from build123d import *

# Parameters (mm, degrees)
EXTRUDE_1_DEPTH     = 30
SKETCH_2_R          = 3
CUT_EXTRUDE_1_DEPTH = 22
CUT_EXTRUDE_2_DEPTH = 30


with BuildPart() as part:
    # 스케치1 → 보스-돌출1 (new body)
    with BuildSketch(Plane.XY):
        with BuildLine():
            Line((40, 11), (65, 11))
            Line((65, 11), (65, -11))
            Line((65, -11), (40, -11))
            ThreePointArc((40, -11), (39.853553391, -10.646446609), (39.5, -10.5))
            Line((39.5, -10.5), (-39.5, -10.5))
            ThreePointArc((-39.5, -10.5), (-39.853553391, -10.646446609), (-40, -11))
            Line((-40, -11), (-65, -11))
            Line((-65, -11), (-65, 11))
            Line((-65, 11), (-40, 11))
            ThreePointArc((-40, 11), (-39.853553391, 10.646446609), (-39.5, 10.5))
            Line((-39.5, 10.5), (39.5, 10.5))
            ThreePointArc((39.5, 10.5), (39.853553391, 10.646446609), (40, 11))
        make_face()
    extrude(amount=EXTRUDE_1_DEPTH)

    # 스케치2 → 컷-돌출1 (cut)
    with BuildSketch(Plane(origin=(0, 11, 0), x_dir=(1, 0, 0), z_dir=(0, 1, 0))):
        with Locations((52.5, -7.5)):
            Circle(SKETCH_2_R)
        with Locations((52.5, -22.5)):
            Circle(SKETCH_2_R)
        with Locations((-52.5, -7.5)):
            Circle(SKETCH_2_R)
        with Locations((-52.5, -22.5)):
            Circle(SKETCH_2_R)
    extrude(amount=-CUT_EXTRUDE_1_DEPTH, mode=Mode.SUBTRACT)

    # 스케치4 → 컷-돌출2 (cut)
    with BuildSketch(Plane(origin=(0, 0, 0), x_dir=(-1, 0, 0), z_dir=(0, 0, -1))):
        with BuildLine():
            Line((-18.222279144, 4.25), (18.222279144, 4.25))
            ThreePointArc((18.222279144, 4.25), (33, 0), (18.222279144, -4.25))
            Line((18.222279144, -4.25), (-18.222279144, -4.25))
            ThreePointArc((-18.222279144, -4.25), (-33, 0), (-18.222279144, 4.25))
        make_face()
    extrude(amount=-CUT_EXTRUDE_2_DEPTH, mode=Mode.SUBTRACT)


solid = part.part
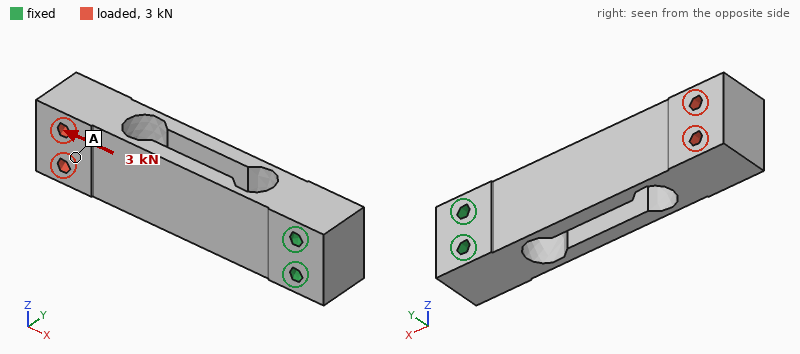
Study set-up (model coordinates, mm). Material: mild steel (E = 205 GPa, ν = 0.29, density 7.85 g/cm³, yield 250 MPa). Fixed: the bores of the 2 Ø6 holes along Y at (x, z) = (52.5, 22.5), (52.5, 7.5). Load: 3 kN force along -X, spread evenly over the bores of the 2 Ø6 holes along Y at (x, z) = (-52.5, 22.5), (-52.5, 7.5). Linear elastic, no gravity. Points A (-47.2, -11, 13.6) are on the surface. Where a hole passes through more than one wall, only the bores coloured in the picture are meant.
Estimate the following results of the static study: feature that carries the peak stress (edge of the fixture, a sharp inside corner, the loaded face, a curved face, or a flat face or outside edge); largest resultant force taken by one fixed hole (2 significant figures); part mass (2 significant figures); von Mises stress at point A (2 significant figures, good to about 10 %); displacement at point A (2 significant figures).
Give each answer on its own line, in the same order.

a curved face
1.5 kN
470 g
4.9 MPa
6.1 µm
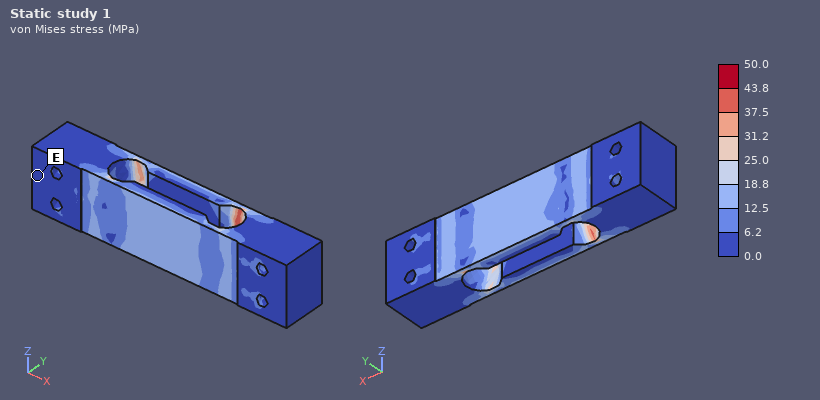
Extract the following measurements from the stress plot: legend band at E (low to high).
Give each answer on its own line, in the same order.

0.0 to 6.2 MPa
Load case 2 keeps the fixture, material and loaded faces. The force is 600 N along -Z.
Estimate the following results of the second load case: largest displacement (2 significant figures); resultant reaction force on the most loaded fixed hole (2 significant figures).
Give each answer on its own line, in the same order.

64 µm
3.4 kN
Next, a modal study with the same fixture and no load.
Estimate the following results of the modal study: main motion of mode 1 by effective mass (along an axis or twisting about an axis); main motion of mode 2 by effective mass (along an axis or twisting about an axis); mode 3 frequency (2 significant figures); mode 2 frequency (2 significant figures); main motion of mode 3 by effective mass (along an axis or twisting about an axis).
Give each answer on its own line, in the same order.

along Y
along Z
2600 Hz
1300 Hz
twisting about X
